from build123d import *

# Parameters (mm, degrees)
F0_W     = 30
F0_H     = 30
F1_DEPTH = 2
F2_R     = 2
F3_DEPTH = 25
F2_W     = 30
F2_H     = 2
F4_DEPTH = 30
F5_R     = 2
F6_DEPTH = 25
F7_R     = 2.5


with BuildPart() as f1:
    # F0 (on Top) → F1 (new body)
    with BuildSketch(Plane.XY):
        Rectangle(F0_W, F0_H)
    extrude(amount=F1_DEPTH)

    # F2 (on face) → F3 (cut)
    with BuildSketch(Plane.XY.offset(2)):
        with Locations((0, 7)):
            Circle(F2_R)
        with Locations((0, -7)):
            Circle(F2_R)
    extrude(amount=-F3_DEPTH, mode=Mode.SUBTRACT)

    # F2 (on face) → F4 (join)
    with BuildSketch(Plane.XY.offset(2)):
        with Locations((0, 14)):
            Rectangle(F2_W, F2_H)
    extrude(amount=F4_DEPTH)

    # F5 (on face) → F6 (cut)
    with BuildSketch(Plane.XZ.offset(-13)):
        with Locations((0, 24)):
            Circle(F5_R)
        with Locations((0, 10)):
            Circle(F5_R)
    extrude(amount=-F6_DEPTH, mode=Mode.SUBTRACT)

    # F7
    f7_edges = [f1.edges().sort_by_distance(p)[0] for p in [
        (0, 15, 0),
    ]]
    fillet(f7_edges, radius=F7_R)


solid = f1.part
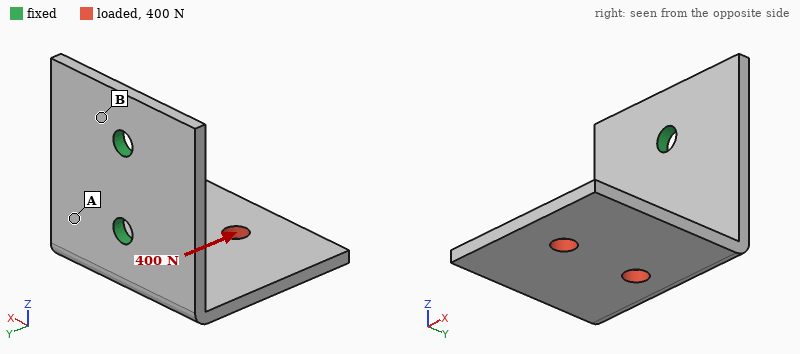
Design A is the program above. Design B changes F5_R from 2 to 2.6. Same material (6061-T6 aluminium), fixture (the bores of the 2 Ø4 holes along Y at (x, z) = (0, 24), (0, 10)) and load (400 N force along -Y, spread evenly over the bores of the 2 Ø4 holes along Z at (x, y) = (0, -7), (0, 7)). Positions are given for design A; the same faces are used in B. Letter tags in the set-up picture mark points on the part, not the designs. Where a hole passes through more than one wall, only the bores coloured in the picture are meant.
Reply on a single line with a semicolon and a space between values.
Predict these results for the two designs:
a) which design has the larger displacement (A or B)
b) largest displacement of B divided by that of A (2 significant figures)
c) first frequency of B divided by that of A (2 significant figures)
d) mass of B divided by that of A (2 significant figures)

A; 0.84; 1.0; 0.99
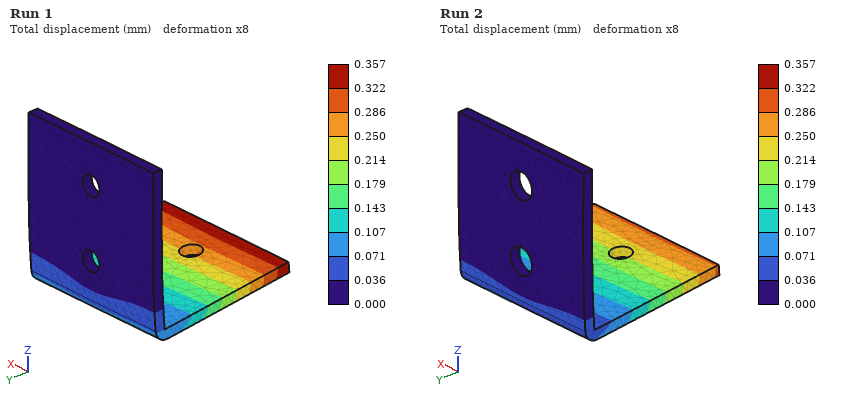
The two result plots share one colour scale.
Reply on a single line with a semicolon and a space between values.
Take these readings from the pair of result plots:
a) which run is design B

Run 2
